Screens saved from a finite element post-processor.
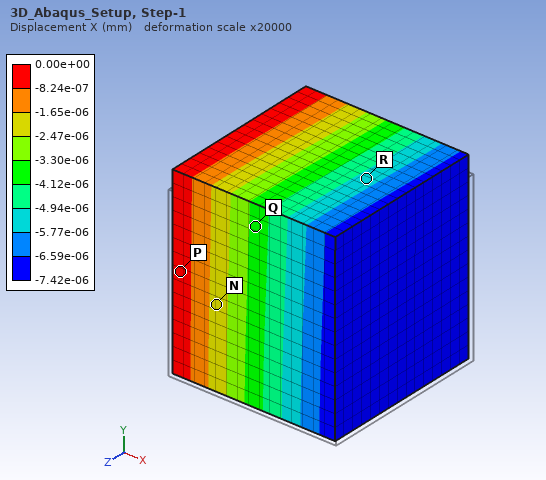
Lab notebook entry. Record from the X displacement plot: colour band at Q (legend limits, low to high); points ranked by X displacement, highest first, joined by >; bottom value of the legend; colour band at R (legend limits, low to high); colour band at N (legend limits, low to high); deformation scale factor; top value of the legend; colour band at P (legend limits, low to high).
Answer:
-4.12e-06 to -3.30e-06 mm
P > N > Q > R
-7.42e-06 mm
-5.77e-06 to -4.94e-06 mm
-2.47e-06 to -1.65e-06 mm
20000
0.00e+00 mm
-8.24e-07 to 0.00e+00 mm
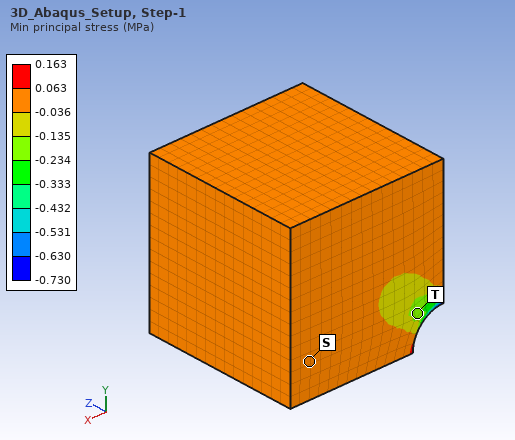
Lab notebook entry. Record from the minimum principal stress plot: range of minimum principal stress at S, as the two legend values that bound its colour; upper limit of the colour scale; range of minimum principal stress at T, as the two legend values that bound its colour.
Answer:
-0.036 to 0.063 MPa
0.163 MPa
-0.234 to -0.135 MPa
